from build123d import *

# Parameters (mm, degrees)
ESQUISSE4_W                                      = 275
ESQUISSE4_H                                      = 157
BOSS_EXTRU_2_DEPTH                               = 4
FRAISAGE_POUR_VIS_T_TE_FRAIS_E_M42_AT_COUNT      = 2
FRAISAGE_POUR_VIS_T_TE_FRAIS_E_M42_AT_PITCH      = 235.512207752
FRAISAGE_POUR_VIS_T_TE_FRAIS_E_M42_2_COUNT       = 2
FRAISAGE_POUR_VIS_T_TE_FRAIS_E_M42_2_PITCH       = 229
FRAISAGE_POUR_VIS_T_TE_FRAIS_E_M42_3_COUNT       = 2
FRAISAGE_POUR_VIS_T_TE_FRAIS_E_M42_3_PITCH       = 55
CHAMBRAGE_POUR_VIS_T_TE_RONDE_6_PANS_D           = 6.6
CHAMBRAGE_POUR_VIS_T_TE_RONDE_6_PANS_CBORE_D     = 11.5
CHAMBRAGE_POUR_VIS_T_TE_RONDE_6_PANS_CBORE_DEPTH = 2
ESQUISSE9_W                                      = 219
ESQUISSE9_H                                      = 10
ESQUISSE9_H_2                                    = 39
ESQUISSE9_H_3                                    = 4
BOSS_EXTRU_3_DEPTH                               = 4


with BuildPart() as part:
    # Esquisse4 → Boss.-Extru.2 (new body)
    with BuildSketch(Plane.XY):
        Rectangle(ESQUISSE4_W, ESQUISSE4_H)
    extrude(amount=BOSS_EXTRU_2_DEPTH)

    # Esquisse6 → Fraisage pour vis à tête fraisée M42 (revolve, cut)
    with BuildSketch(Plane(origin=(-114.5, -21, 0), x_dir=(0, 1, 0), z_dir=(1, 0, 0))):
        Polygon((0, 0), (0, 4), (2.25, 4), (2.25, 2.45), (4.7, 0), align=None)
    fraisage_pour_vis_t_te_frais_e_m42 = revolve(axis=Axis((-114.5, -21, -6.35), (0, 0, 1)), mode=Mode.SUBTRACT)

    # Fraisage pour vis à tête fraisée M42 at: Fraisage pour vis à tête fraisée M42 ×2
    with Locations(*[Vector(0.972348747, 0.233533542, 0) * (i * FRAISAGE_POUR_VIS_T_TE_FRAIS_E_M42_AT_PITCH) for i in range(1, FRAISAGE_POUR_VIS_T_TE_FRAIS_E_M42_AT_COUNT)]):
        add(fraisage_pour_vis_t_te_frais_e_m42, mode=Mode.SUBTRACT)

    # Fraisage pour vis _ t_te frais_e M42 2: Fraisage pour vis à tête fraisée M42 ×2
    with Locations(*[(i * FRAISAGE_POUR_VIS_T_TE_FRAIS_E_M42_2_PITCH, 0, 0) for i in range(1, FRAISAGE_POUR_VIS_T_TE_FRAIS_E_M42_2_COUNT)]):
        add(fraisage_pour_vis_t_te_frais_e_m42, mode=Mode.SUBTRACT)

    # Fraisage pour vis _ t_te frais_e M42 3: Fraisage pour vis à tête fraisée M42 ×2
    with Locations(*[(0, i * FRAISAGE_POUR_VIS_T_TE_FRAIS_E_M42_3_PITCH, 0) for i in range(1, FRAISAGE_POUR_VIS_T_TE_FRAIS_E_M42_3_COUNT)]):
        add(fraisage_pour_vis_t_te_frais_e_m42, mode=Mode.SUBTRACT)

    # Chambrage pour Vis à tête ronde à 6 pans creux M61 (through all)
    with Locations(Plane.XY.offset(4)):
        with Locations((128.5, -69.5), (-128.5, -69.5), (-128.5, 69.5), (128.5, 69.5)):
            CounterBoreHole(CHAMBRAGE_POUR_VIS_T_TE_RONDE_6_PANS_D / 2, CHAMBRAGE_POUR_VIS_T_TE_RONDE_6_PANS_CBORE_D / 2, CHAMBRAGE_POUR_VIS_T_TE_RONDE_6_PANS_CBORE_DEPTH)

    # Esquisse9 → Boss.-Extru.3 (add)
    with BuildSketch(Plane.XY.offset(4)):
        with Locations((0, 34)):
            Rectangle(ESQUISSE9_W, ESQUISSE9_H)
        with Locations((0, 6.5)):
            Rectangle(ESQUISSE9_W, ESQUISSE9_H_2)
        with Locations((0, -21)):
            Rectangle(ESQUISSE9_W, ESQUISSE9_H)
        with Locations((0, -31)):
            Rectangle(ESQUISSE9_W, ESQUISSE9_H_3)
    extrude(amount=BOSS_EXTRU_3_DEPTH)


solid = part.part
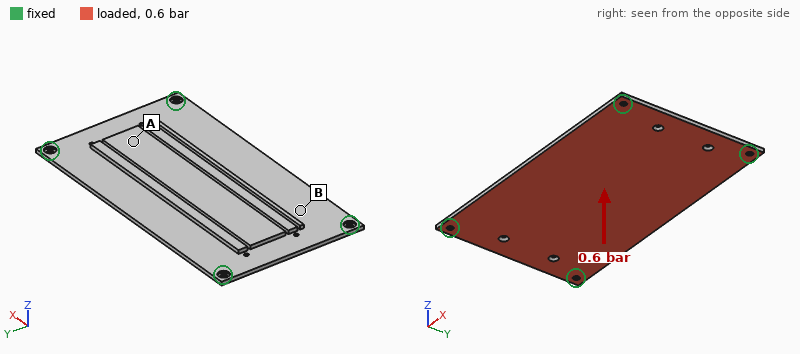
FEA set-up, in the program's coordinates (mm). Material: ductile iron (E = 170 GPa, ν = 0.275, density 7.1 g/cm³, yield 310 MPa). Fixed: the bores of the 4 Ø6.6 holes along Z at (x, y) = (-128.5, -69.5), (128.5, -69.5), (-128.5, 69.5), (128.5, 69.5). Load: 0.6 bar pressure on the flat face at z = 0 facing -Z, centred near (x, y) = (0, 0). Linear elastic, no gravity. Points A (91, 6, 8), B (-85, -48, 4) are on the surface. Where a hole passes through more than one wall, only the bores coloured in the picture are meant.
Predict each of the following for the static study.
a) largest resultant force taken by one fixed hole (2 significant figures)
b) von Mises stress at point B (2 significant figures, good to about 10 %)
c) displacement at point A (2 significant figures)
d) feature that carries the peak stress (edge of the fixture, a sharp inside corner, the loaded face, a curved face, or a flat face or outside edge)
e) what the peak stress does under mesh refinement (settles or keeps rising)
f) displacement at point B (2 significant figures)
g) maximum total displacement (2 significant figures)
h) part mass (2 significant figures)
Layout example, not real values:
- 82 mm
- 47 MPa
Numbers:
- 2.9 kN
- 49 MPa
- 0.32 mm
- edge of the fixture
- keeps rising
- 0.33 mm
- 0.68 mm
- 1.6 kg
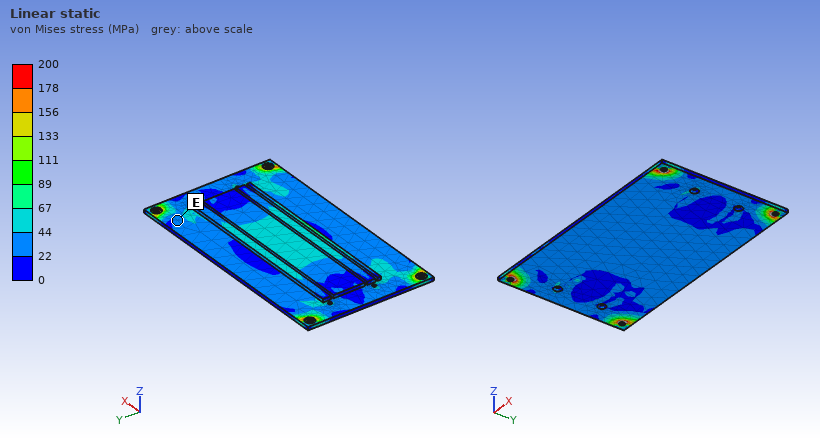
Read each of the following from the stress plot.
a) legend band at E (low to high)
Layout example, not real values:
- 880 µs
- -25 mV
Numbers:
- 22 to 44 MPa
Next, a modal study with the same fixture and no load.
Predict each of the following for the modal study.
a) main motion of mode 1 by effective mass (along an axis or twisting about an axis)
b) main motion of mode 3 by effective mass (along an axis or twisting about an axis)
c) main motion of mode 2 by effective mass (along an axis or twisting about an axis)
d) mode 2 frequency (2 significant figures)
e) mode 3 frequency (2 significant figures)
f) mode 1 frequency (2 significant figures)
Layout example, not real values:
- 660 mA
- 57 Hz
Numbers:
- along Z
- twisting about Y
- twisting about X
- 540 Hz
- 710 Hz
- 290 Hz
